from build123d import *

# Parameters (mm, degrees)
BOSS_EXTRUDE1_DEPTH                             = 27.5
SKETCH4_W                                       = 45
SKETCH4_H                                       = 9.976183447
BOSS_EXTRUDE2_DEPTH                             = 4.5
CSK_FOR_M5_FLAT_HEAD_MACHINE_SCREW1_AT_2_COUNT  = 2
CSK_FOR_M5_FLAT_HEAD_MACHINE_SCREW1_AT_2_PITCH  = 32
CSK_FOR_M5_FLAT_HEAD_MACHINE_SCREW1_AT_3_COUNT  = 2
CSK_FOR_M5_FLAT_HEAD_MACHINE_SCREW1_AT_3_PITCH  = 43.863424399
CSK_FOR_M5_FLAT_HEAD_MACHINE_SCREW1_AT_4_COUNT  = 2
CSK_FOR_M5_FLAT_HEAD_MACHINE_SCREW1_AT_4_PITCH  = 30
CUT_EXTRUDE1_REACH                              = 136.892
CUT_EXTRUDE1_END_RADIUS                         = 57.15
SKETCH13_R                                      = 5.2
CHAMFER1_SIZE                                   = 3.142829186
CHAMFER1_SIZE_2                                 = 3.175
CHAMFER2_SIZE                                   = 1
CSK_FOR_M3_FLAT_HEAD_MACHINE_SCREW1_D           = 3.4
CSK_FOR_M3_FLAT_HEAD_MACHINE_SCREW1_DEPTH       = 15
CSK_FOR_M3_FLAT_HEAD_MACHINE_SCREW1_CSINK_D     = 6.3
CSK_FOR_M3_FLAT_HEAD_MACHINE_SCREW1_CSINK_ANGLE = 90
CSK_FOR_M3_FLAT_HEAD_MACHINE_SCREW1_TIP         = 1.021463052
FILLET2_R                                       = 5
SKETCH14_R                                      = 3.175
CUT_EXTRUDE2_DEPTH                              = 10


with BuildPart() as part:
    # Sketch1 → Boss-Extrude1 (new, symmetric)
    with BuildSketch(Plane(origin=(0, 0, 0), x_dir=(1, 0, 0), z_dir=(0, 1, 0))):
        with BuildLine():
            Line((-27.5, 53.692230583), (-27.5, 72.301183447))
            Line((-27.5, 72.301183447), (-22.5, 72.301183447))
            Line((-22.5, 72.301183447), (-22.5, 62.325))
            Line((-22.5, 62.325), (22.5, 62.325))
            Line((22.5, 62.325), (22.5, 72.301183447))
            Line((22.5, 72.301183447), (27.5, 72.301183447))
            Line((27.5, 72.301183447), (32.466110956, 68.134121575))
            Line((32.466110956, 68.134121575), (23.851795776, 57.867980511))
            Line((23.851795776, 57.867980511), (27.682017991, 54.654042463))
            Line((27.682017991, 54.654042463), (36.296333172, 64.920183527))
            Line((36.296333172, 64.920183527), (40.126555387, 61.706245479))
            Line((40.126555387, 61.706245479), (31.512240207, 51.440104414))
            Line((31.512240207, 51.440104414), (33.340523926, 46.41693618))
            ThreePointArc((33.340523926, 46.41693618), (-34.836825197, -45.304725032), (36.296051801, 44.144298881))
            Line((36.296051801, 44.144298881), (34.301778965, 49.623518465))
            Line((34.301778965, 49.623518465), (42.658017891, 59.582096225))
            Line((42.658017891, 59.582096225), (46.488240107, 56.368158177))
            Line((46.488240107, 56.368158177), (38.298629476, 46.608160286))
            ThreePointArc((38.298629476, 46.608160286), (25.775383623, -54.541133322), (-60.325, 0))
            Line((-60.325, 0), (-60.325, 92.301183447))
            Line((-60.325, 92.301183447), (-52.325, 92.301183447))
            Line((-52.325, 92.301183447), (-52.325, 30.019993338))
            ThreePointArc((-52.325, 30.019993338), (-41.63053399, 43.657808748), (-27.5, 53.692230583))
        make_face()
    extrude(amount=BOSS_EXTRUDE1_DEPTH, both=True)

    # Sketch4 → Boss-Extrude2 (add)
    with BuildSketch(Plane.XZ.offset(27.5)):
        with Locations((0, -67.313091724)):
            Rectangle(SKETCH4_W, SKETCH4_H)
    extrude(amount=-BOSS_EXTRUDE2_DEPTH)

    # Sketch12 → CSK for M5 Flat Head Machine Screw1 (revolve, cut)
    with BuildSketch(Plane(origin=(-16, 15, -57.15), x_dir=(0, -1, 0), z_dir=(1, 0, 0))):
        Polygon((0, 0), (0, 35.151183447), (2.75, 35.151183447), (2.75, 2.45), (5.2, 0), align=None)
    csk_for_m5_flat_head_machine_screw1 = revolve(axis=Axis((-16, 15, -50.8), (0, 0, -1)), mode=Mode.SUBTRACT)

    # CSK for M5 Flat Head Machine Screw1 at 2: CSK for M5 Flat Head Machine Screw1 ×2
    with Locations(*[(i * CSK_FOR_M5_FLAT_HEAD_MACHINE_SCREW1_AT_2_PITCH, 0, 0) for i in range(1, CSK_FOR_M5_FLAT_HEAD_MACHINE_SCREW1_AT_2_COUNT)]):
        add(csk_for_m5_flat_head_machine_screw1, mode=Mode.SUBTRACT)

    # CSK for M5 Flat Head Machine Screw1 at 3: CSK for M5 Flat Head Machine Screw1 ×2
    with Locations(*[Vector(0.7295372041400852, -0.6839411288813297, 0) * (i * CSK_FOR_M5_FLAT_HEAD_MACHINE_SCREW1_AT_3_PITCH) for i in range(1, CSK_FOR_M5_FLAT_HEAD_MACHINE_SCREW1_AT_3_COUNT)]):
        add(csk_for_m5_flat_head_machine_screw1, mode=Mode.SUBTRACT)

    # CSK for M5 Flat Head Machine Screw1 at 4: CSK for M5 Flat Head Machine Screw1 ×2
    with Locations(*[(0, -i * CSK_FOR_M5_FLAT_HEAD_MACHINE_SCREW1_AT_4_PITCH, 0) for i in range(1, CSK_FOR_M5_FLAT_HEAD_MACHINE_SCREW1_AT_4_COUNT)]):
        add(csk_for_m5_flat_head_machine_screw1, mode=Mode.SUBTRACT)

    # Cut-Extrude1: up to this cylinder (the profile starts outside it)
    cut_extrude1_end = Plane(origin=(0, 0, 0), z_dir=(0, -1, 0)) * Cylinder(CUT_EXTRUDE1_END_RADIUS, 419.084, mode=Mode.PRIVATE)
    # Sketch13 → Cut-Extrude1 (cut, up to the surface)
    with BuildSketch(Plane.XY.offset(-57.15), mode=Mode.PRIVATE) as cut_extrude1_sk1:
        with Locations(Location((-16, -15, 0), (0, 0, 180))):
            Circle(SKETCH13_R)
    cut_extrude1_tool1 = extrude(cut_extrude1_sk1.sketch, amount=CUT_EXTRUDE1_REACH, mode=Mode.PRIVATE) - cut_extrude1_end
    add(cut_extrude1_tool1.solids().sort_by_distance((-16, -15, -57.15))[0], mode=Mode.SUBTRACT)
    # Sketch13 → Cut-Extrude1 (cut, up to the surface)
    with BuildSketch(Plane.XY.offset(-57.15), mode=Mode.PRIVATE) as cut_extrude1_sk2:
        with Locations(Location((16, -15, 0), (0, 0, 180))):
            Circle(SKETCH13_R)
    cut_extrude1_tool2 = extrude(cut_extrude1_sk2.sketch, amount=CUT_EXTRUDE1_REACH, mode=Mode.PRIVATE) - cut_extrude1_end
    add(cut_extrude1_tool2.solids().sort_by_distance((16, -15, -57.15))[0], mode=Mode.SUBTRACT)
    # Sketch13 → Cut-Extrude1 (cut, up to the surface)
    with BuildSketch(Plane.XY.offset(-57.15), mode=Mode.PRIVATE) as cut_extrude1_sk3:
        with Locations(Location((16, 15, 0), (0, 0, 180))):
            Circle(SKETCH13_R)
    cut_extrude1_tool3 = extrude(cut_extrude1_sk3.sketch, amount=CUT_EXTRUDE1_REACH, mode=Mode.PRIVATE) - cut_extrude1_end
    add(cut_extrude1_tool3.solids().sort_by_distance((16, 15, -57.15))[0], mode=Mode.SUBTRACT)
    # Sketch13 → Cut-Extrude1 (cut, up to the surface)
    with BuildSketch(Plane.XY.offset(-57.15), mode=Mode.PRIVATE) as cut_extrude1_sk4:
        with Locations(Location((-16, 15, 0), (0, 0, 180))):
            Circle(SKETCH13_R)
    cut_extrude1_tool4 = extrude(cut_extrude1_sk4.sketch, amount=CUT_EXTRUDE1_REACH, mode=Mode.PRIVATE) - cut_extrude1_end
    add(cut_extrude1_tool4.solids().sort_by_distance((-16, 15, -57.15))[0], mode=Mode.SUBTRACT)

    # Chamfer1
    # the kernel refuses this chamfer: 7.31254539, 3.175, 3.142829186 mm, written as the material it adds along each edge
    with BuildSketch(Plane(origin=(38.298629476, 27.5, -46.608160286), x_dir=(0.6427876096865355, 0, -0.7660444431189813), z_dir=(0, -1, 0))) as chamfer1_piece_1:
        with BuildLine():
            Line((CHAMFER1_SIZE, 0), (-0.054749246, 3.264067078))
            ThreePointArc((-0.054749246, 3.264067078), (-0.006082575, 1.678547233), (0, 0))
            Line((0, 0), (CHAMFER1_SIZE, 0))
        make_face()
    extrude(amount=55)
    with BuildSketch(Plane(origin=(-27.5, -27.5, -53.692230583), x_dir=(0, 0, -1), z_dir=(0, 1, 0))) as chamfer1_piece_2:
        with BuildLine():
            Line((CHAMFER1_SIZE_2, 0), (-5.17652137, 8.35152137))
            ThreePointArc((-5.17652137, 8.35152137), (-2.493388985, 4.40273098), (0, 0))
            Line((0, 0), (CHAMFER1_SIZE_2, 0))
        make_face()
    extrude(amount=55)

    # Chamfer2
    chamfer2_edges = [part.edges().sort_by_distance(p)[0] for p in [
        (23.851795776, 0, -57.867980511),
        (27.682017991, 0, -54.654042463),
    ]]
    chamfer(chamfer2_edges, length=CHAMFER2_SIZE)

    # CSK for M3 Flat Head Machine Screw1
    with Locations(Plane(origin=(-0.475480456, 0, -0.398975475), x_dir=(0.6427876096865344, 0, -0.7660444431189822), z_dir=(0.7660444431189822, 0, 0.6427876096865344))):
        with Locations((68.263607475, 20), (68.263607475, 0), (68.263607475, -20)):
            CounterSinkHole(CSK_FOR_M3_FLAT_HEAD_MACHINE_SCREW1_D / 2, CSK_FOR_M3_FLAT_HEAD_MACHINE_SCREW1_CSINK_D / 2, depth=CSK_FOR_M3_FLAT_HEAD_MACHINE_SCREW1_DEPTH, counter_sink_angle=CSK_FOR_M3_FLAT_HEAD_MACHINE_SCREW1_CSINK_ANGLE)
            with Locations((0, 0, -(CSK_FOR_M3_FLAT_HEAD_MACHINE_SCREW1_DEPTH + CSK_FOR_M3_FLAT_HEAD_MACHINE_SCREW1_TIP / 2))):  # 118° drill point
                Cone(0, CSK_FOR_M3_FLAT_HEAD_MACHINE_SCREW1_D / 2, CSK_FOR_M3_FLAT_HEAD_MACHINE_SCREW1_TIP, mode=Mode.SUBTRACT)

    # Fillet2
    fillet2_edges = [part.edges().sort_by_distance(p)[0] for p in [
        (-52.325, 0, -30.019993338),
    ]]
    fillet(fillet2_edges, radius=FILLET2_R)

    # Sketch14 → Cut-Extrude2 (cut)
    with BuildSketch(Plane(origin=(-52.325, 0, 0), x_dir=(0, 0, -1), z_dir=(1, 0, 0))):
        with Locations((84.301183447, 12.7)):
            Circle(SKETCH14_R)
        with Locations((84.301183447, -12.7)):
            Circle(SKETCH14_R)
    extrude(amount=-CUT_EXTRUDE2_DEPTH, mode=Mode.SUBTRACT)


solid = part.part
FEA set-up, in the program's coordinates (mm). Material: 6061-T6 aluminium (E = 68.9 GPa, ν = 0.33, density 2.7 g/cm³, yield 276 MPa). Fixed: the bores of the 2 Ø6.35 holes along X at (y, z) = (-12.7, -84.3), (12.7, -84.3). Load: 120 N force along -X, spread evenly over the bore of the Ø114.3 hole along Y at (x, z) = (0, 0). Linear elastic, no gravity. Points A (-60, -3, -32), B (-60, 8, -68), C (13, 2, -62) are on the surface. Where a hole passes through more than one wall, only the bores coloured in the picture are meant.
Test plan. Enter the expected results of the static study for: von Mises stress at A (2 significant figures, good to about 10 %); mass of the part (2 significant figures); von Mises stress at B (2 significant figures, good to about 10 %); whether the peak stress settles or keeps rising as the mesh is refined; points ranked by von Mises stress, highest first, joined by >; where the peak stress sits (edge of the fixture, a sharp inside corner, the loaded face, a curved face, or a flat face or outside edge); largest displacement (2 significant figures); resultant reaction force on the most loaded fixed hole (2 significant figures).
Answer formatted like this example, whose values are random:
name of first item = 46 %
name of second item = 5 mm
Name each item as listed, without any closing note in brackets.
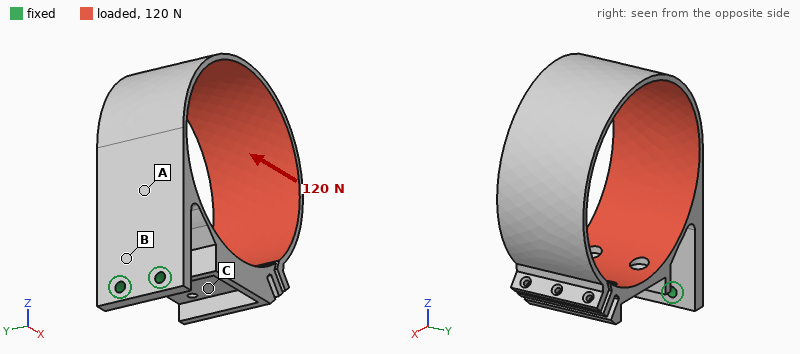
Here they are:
von Mises stress at A = 4.5 MPa
mass of the part = 340 g
von Mises stress at B = 13 MPa
whether the peak stress settles or keeps rising as the mesh is refined = keeps rising
points ranked by von Mises stress, highest first, joined by > = B > A > C
where the peak stress sits = edge of the fixture
largest displacement = 2.0 mm
resultant reaction force on the most loaded fixed hole = 60 N
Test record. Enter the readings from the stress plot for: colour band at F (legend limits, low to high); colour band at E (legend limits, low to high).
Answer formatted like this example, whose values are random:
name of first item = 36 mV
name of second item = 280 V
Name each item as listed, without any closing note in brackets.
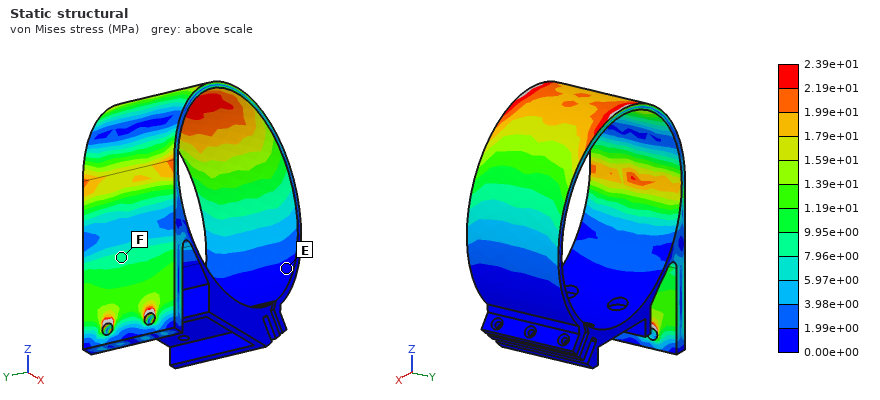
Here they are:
colour band at F = 7.96e+00 to 9.95e+00 MPa
colour band at E = 0.00e+00 to 1.99e+00 MPa
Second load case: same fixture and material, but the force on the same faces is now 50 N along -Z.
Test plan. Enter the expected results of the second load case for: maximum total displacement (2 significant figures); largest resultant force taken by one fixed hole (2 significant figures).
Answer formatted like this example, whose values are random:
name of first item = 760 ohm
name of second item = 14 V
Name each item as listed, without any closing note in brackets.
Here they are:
maximum total displacement = 2.3 mm
largest resultant force taken by one fixed hole = 25 N
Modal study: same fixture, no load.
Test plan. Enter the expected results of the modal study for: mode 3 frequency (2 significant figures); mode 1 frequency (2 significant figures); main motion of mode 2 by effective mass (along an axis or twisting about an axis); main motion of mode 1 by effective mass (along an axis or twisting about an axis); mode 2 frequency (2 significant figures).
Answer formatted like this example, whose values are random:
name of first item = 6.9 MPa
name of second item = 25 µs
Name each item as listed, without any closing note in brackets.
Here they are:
mode 3 frequency = 120 Hz
mode 1 frequency = 55 Hz
main motion of mode 2 by effective mass = along Y
main motion of mode 1 by effective mass = along Z
mode 2 frequency = 73 Hz
